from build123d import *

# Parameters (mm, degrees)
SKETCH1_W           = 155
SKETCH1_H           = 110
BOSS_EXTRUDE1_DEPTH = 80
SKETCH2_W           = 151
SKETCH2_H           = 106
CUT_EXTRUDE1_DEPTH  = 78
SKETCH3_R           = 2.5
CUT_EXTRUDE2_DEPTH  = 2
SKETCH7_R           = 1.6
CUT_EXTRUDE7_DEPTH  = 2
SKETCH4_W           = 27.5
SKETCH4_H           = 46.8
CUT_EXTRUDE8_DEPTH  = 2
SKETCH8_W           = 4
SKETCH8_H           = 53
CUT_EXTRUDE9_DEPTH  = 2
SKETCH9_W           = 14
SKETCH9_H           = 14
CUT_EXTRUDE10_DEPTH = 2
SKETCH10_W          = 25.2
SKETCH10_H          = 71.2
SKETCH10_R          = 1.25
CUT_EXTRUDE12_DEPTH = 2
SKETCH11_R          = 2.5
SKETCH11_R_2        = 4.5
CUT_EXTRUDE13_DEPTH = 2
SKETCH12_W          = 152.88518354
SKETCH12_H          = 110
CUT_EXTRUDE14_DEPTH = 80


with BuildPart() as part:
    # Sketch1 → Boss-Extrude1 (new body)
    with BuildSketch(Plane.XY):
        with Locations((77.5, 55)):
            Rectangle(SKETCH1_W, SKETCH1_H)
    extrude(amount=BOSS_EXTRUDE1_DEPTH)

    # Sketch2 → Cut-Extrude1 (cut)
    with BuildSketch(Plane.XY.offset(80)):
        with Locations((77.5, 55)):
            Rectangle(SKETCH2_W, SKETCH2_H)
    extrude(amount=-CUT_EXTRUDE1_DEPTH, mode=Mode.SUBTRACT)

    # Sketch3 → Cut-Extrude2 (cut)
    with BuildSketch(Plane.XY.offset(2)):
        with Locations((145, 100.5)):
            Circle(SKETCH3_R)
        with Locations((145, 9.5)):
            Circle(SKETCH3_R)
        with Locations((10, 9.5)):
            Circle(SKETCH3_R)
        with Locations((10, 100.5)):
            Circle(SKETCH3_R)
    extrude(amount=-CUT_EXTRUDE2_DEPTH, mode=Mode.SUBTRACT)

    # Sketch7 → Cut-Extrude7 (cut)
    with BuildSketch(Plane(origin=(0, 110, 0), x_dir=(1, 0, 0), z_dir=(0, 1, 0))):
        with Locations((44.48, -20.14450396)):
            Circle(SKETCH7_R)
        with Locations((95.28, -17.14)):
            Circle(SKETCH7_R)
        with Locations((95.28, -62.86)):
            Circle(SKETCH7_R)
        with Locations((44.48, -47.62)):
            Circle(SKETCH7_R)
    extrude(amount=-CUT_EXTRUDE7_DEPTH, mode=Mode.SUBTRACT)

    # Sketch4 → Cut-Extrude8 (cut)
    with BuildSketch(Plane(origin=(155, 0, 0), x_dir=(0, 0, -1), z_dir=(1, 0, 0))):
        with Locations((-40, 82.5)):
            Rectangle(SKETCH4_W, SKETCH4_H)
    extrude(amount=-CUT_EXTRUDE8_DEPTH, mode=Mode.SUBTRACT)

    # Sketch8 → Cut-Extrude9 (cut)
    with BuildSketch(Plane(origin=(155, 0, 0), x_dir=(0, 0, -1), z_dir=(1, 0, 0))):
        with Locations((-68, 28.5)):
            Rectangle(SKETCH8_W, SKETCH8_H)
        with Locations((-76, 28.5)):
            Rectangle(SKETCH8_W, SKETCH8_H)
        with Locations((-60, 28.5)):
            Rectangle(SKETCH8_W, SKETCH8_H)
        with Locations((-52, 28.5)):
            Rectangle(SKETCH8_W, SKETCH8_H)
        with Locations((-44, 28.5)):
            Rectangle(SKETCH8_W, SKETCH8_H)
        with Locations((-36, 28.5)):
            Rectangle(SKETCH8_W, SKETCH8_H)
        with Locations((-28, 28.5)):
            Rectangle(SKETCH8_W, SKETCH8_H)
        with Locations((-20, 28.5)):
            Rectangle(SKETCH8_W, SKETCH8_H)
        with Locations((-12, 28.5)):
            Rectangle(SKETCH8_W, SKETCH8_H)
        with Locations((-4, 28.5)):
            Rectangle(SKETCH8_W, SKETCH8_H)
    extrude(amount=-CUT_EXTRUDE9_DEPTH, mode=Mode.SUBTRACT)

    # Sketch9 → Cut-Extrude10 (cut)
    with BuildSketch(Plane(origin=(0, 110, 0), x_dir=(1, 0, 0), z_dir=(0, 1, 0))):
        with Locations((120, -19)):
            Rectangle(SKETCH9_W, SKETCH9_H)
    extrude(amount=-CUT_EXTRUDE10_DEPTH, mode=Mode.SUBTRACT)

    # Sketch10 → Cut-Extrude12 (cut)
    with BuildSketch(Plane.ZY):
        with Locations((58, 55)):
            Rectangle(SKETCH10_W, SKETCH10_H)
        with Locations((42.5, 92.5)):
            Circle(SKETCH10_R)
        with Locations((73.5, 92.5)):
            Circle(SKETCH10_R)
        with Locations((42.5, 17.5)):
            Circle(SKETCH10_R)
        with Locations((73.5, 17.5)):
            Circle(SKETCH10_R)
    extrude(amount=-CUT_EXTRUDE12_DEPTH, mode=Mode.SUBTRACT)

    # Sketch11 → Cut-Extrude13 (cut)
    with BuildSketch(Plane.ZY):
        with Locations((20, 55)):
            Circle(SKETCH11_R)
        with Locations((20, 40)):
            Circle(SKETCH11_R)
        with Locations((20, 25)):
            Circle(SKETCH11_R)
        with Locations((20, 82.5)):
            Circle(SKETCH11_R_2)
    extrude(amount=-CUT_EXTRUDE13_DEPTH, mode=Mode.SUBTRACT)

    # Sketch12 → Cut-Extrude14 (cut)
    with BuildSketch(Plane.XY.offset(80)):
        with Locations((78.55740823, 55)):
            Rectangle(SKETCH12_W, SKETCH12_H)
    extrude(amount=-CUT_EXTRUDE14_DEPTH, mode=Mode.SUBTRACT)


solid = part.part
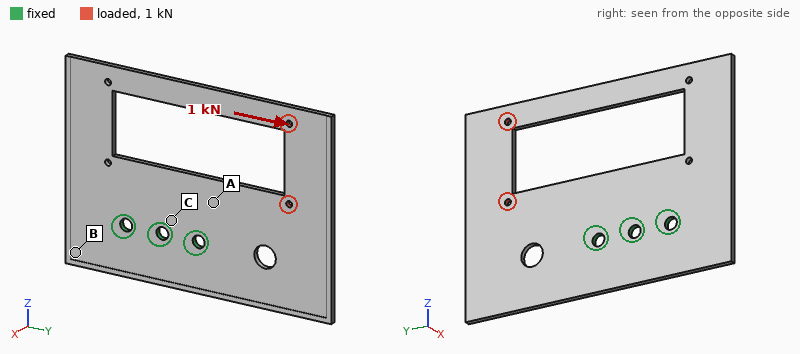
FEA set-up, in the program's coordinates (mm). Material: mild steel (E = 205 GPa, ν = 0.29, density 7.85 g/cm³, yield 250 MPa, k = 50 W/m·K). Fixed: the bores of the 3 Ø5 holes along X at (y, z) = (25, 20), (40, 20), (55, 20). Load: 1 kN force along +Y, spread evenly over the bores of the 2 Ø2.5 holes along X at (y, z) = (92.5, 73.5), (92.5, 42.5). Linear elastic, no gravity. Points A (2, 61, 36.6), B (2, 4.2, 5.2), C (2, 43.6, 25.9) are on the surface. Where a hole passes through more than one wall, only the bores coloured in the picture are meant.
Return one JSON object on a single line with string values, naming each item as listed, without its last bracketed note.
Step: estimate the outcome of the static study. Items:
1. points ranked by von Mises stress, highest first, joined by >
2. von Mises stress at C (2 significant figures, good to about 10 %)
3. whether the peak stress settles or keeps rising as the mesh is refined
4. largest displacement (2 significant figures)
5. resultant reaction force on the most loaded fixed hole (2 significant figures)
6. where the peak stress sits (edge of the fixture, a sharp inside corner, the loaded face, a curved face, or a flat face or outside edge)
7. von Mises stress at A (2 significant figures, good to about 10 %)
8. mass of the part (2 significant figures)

{"points ranked by von Mises stress, highest first, joined by >": "C > A > B", "von Mises stress at C": "37 MPa", "whether the peak stress settles or keeps rising as the mesh is refined": "keeps rising", "largest displacement": "54 µm", "resultant reaction force on the most loaded fixed hole": "1.2 kN", "where the peak stress sits": "a sharp inside corner", "von Mises stress at A": "25 MPa", "mass of the part": "110 g"}
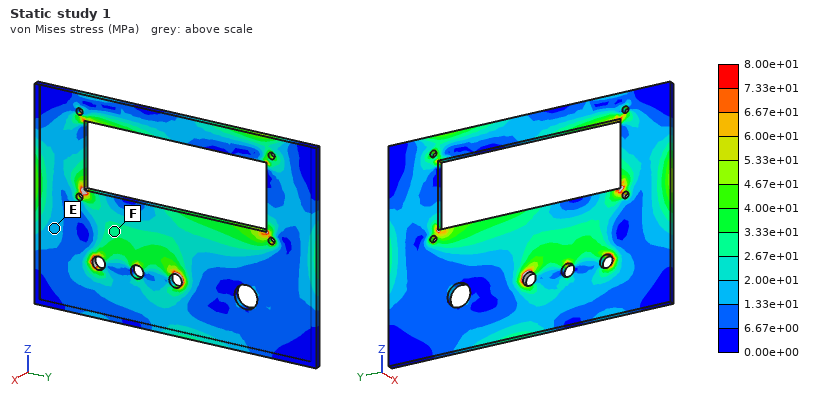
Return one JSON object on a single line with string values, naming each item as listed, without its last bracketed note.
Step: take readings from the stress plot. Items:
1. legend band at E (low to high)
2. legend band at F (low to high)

{"legend band at E": "1.33e+01 to 2.00e+01 MPa", "legend band at F": "2.67e+01 to 3.33e+01 MPa"}
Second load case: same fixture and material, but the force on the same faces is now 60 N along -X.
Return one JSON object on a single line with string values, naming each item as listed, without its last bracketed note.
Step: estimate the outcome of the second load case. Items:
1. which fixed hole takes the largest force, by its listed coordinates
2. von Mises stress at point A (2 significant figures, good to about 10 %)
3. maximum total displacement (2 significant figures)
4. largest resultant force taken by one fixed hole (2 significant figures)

{"which fixed hole takes the largest force, by its listed coordinates": "(55, 20)", "von Mises stress at point A": "67 MPa", "maximum total displacement": "0.94 mm", "largest resultant force taken by one fixed hole": "110 N"}
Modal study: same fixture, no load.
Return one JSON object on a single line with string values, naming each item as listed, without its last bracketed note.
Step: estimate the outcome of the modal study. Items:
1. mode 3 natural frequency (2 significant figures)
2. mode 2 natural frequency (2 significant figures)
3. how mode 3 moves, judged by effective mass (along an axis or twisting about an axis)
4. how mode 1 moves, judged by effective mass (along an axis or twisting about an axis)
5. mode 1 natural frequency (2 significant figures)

{"mode 3 natural frequency": "700 Hz", "mode 2 natural frequency": "460 Hz", "how mode 3 moves, judged by effective mass": "along X", "how mode 1 moves, judged by effective mass": "along X", "mode 1 natural frequency": "310 Hz"}
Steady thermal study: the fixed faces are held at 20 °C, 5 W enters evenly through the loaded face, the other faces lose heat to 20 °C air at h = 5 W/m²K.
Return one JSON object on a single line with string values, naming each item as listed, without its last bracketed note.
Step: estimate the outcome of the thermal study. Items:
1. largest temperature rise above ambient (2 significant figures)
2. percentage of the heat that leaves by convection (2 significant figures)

{"largest temperature rise above ambient": "74 K", "percentage of the heat that leaves by convection": "30 %"}
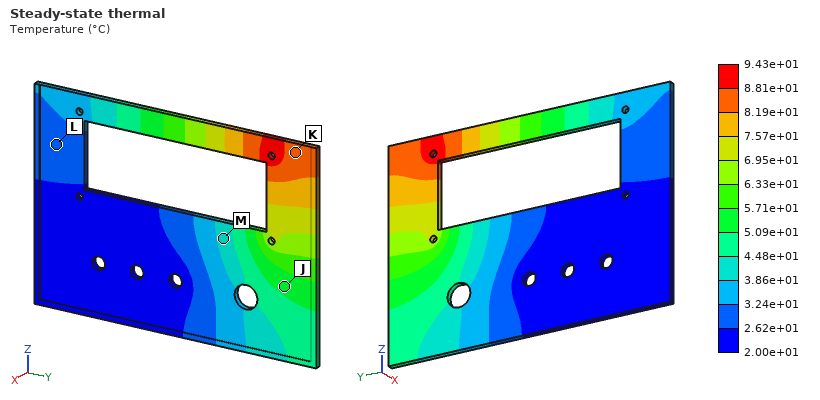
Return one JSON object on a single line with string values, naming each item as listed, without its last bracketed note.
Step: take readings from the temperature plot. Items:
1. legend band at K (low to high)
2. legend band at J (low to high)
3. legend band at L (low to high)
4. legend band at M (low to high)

{"legend band at K": "8.19e+01 to 8.81e+01 °C", "legend band at J": "5.09e+01 to 5.71e+01 °C", "legend band at L": "2.62e+01 to 3.24e+01 °C", "legend band at M": "3.86e+01 to 4.48e+01 °C"}
